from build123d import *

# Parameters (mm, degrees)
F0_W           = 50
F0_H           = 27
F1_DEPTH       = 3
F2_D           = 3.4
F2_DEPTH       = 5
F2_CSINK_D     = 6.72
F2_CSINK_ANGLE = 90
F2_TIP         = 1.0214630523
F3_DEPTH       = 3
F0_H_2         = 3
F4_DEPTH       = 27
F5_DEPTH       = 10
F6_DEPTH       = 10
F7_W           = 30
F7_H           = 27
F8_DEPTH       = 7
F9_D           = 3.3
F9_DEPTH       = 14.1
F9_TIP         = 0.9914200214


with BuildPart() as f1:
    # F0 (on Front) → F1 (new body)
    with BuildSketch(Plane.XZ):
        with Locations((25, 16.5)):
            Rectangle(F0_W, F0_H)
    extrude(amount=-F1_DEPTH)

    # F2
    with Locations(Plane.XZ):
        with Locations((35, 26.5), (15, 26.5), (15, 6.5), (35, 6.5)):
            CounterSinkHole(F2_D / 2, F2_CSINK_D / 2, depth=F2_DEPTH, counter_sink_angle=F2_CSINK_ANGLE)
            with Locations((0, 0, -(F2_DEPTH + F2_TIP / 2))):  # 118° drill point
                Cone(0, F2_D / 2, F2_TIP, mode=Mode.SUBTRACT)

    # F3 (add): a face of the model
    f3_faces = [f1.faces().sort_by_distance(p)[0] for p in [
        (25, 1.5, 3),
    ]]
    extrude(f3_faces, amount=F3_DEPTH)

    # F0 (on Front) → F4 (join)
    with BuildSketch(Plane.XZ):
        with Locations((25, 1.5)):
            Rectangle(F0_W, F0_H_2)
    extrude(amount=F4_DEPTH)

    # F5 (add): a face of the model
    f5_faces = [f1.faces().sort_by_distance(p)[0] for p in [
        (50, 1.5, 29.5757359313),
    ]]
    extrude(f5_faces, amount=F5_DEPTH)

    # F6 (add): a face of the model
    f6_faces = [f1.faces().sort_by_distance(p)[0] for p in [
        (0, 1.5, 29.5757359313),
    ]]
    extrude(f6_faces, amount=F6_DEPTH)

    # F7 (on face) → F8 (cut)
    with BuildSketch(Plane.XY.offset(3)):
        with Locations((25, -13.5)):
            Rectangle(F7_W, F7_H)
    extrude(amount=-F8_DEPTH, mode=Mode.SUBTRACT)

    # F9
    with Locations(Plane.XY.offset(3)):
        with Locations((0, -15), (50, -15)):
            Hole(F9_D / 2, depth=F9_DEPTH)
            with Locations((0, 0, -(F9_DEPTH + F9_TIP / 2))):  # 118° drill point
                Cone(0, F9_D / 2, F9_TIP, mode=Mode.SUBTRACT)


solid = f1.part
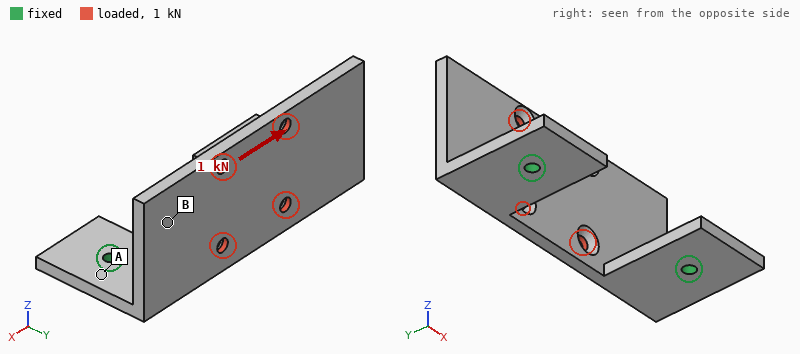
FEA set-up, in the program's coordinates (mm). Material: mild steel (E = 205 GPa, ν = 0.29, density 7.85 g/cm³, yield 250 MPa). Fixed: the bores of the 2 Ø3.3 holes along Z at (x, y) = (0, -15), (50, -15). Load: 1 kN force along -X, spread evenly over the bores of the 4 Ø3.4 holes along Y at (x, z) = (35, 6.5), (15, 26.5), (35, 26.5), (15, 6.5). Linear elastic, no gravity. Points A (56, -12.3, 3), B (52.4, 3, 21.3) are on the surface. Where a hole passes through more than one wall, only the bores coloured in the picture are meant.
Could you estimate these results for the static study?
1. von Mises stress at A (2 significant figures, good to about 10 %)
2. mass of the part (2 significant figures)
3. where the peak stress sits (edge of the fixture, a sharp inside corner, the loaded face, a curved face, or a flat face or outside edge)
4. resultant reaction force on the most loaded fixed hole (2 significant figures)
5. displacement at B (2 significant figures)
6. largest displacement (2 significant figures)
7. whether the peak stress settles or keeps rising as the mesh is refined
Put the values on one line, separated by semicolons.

50 MPa; 73 g; edge of the fixture; 580 N; 51 µm; 67 µm; keeps rising
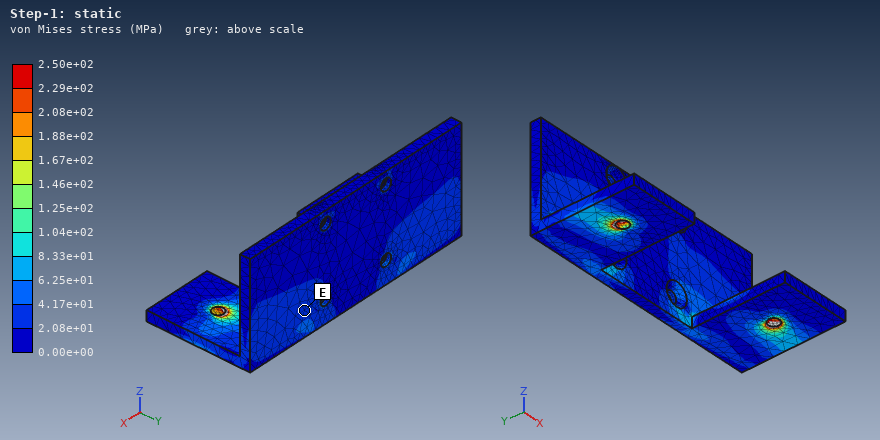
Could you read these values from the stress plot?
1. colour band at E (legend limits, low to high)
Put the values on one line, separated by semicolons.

2.08e+01 to 4.17e+01 MPa
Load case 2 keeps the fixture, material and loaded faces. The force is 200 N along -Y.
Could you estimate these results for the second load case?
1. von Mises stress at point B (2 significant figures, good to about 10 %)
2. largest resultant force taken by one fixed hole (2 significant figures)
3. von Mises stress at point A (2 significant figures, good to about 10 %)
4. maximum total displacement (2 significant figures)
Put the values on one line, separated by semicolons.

11 MPa; 120 N; 39 MPa; 0.12 mm
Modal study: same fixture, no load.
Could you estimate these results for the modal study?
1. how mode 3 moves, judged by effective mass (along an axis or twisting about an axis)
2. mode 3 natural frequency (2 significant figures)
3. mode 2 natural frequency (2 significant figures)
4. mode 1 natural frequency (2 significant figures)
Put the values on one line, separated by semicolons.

along Z; 3800 Hz; 2400 Hz; 1200 Hz
